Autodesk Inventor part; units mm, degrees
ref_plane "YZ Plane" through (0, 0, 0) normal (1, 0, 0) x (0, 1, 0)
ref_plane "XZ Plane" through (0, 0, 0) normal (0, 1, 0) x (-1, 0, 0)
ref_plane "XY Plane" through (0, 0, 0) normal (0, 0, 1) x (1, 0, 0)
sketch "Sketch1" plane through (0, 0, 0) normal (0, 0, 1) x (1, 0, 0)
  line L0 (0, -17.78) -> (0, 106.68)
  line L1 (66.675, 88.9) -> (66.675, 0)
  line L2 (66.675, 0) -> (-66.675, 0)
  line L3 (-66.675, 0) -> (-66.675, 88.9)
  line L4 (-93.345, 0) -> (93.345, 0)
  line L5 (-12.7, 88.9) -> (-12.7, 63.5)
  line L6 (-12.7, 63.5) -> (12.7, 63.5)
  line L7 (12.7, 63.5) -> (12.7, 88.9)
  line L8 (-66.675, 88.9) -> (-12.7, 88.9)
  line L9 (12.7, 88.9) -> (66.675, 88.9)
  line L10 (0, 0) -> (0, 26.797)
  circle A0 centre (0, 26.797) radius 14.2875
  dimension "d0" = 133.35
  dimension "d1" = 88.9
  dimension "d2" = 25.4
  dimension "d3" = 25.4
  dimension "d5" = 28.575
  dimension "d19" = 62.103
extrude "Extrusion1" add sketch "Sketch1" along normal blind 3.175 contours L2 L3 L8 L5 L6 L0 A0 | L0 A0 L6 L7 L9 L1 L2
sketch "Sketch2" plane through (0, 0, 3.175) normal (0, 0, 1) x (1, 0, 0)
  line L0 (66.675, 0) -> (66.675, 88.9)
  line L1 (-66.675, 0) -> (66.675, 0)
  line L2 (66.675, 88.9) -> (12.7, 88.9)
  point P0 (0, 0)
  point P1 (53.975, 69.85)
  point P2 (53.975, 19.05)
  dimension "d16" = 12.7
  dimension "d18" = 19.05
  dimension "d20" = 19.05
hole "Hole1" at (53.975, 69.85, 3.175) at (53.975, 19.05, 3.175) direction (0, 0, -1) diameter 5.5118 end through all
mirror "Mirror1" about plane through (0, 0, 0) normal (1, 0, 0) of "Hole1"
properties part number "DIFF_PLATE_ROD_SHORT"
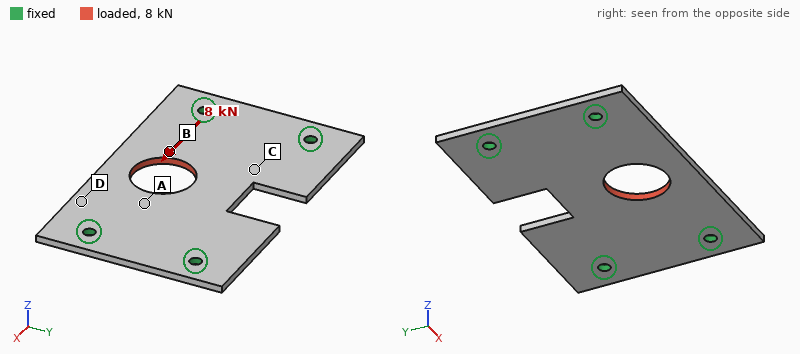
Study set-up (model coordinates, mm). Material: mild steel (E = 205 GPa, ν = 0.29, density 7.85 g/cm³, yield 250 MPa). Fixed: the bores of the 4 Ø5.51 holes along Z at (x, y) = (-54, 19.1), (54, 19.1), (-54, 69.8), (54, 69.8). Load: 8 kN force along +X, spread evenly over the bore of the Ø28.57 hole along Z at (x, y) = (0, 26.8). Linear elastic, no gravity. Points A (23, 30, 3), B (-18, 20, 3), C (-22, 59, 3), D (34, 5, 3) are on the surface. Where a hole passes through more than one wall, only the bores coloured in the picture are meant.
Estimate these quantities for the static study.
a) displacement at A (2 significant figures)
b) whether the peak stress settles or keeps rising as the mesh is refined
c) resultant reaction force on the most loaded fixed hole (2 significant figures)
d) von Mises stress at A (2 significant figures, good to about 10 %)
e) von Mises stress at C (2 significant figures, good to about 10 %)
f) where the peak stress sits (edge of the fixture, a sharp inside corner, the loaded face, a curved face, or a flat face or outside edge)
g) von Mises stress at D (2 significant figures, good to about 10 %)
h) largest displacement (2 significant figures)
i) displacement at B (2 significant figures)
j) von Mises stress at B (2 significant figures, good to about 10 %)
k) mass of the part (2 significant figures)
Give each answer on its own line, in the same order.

4.9 µm
keeps rising
2.8 kN
27 MPa
12 MPa
edge of the fixture
18 MPa
8.2 µm
6.0 µm
33 MPa
260 g
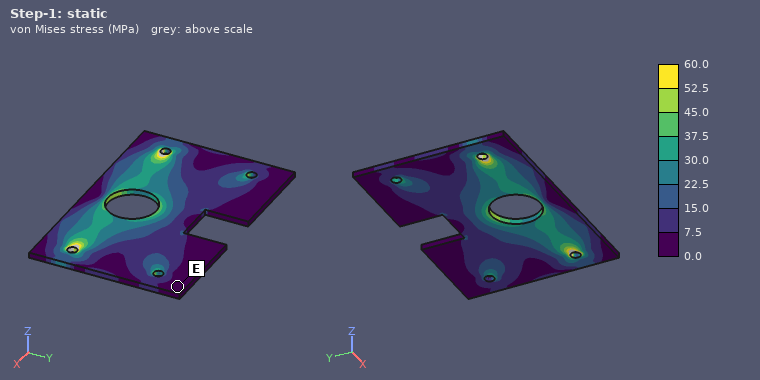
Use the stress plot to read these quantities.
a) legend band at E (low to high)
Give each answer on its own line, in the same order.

0.0 to 7.5 MPa
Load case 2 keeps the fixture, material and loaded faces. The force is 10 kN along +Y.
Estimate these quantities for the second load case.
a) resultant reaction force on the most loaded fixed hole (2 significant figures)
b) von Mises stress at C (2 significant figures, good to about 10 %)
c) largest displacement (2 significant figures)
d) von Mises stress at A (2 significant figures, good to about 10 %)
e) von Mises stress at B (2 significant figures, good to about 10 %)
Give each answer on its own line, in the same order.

3.8 kN
30 MPa
26 µm
60 MPa
59 MPa
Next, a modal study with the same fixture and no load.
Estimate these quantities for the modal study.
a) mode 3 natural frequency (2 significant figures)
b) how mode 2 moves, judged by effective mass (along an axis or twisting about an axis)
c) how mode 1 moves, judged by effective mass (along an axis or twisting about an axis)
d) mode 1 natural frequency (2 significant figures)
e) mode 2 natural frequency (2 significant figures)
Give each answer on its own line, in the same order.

2800 Hz
twisting about X
along Z
1400 Hz
1900 Hz
